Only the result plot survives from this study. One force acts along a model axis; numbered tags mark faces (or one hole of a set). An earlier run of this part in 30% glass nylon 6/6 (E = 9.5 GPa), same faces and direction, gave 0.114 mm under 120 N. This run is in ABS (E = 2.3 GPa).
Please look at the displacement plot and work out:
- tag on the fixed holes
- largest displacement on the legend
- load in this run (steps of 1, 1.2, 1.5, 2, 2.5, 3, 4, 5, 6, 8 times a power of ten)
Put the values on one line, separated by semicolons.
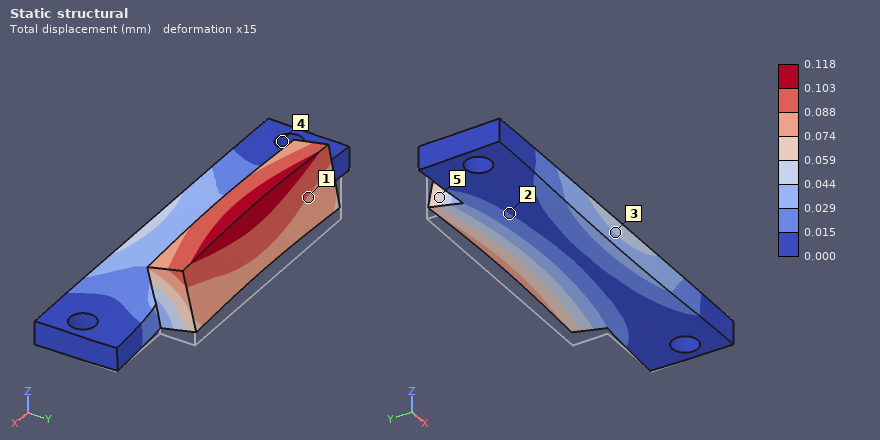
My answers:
4; 0.118 mm; 30 N
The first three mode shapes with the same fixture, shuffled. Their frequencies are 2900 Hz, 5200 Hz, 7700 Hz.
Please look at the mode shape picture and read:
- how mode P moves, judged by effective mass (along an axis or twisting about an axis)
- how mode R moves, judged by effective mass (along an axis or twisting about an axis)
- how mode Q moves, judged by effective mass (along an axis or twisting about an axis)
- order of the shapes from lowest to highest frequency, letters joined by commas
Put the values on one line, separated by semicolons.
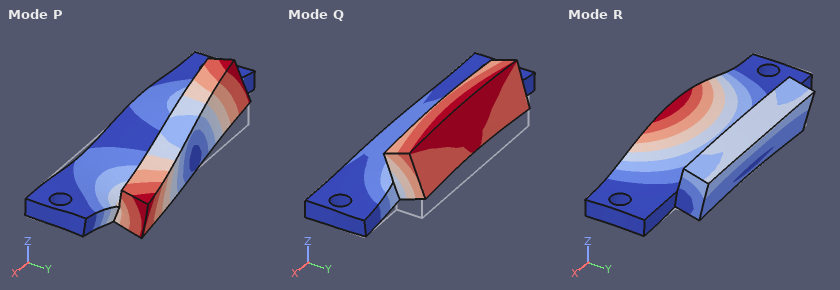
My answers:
twisting about Y; along Z; along Z; Q, R, P
